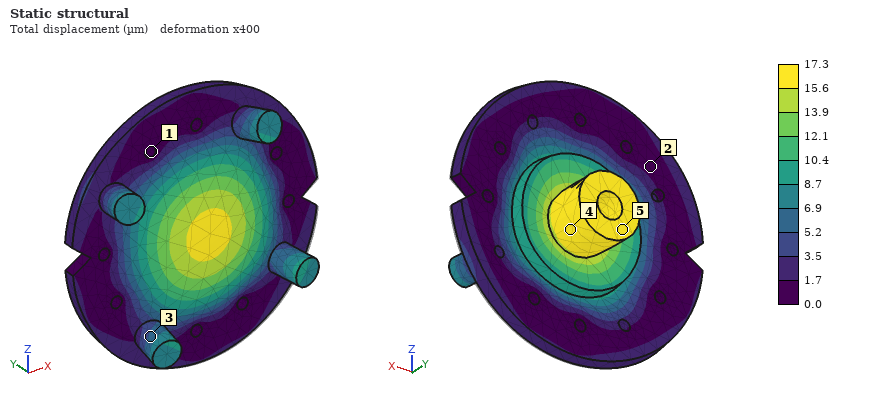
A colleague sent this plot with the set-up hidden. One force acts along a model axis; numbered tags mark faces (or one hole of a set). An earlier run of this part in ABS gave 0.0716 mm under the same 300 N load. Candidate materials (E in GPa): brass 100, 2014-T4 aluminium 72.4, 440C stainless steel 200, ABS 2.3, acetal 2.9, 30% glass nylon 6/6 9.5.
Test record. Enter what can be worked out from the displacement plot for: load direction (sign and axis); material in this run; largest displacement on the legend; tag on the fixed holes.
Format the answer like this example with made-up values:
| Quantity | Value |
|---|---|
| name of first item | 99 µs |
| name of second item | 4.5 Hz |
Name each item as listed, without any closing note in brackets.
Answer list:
| Quantity | Value |
|---|---|
| load direction | -Y |
| material in this run | 30% glass nylon 6/6 |
| largest displacement on the legend | 17.3 µm |
| tag on the fixed holes | 1 |
